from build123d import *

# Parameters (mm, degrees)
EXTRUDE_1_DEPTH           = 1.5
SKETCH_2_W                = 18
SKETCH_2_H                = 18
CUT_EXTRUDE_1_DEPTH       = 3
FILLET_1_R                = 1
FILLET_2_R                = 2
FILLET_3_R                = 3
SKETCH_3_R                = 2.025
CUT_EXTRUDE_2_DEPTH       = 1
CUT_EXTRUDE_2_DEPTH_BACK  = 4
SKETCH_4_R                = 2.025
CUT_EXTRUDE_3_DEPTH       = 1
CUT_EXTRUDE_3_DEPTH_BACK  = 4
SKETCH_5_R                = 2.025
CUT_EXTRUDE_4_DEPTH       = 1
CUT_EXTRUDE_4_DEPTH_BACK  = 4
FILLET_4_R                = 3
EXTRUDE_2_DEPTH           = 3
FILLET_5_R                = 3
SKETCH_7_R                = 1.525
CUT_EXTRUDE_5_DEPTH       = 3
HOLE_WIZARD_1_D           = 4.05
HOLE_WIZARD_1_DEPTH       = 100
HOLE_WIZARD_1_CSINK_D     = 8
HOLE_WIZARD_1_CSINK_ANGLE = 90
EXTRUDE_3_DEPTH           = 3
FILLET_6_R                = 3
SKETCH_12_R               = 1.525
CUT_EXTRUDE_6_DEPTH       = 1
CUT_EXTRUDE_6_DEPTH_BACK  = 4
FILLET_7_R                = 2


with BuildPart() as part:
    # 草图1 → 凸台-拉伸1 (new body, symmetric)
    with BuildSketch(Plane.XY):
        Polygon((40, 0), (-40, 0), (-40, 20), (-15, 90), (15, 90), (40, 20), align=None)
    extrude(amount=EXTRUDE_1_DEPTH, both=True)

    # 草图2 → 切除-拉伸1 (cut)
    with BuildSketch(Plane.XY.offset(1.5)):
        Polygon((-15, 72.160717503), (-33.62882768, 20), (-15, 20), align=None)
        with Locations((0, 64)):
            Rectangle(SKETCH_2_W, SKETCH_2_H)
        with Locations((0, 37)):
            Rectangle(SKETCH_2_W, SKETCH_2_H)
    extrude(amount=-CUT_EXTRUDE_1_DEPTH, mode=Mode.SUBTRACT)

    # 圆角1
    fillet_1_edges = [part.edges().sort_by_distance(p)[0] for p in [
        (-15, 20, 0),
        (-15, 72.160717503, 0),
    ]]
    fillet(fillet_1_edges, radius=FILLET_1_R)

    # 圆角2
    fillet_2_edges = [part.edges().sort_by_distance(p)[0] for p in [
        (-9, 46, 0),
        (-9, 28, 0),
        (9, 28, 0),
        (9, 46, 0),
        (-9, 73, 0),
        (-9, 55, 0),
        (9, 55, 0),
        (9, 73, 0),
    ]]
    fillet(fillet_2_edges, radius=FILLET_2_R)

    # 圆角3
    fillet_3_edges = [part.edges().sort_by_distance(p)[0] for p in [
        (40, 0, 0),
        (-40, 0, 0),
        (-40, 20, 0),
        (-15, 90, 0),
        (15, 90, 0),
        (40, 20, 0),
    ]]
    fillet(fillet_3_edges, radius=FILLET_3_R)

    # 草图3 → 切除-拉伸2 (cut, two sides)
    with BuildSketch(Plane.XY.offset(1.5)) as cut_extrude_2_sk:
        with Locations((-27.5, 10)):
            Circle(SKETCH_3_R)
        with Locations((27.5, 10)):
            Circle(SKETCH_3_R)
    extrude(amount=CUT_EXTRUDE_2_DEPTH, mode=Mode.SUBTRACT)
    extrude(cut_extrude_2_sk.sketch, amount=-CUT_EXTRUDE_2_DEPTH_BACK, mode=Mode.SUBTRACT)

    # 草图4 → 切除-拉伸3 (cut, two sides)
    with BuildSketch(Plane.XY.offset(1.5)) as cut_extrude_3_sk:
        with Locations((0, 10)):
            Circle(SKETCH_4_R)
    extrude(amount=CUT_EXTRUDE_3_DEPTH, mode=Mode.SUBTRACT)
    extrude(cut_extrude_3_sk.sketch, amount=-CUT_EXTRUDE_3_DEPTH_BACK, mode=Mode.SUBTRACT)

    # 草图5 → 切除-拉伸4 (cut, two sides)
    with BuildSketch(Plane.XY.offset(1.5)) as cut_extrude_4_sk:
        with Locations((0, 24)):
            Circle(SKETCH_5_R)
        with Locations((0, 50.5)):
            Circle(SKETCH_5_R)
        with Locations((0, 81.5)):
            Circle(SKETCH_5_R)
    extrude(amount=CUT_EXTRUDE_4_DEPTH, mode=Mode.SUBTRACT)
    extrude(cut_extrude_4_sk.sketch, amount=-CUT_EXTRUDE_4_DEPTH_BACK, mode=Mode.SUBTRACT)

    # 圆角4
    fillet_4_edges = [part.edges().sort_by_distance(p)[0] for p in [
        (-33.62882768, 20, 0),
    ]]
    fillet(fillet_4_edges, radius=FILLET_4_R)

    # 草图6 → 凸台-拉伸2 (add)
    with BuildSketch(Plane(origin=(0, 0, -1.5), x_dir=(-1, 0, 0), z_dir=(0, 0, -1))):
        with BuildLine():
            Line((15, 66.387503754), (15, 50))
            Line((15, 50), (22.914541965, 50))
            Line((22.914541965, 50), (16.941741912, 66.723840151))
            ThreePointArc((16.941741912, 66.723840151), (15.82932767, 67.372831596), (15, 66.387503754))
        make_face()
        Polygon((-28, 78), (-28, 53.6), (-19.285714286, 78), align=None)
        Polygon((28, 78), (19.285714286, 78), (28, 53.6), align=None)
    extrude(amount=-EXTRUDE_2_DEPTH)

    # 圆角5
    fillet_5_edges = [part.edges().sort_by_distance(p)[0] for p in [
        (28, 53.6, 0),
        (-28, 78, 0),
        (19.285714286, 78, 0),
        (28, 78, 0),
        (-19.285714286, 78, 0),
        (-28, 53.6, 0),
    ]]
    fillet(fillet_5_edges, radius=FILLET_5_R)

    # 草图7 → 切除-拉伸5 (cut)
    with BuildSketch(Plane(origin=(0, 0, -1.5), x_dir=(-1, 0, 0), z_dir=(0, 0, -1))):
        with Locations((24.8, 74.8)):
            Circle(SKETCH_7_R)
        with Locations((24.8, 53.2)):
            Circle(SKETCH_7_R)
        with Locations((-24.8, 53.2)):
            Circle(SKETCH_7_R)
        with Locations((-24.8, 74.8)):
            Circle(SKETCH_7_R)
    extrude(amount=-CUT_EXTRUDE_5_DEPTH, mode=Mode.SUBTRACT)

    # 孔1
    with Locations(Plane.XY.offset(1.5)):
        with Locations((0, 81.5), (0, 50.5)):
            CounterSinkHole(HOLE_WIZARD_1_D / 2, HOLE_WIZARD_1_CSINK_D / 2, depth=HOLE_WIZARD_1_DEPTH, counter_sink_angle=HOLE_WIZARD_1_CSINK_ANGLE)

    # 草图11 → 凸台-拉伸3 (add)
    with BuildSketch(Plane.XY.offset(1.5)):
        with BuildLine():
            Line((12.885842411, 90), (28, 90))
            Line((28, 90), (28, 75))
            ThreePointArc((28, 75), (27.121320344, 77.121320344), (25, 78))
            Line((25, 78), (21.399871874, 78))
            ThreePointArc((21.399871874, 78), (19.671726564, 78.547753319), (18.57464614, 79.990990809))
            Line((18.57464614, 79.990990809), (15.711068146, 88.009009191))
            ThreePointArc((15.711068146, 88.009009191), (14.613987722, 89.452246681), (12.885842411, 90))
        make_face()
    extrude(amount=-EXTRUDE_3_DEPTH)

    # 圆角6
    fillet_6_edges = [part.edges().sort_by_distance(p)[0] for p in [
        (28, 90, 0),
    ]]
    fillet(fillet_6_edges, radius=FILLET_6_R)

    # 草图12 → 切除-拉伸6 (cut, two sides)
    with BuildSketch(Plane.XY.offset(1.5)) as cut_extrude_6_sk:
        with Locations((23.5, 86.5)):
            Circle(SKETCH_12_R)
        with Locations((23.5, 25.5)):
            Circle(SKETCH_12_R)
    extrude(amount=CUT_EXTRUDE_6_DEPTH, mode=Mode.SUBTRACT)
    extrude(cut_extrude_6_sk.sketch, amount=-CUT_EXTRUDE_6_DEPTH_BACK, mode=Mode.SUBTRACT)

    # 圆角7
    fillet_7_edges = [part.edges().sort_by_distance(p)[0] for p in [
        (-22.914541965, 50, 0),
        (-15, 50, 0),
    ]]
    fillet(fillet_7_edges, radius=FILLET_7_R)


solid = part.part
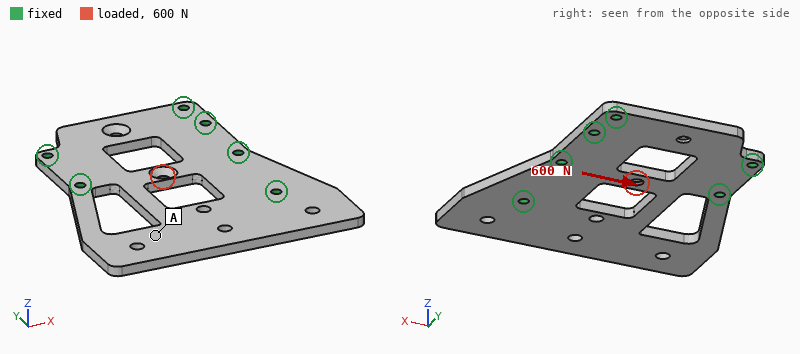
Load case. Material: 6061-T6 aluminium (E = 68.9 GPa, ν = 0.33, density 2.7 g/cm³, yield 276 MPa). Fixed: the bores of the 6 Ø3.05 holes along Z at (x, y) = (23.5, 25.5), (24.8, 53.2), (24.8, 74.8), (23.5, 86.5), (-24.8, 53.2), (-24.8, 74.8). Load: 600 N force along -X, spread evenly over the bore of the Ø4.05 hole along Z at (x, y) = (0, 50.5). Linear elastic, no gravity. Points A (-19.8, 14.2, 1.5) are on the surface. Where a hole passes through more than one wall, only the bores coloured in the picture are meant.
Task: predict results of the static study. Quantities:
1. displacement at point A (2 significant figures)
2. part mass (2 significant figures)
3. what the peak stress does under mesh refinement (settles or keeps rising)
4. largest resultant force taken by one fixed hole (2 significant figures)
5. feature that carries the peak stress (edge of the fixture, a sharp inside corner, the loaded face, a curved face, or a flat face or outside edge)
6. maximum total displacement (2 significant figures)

1.7 µm
37 g
keeps rising
250 N
a sharp inside corner
6.1 µm
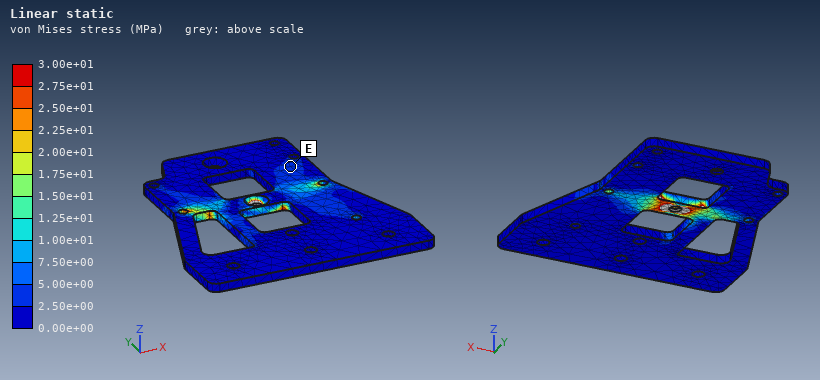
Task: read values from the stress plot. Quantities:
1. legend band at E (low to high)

2.50e+00 to 5.00e+00 MPa
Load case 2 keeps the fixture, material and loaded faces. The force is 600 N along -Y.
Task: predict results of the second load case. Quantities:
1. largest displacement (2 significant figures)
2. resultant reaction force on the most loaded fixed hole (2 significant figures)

18 µm
180 N
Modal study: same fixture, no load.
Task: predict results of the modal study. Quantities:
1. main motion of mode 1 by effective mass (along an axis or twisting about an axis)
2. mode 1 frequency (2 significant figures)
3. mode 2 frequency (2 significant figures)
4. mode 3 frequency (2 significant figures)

along Z
980 Hz
2900 Hz
4000 Hz
